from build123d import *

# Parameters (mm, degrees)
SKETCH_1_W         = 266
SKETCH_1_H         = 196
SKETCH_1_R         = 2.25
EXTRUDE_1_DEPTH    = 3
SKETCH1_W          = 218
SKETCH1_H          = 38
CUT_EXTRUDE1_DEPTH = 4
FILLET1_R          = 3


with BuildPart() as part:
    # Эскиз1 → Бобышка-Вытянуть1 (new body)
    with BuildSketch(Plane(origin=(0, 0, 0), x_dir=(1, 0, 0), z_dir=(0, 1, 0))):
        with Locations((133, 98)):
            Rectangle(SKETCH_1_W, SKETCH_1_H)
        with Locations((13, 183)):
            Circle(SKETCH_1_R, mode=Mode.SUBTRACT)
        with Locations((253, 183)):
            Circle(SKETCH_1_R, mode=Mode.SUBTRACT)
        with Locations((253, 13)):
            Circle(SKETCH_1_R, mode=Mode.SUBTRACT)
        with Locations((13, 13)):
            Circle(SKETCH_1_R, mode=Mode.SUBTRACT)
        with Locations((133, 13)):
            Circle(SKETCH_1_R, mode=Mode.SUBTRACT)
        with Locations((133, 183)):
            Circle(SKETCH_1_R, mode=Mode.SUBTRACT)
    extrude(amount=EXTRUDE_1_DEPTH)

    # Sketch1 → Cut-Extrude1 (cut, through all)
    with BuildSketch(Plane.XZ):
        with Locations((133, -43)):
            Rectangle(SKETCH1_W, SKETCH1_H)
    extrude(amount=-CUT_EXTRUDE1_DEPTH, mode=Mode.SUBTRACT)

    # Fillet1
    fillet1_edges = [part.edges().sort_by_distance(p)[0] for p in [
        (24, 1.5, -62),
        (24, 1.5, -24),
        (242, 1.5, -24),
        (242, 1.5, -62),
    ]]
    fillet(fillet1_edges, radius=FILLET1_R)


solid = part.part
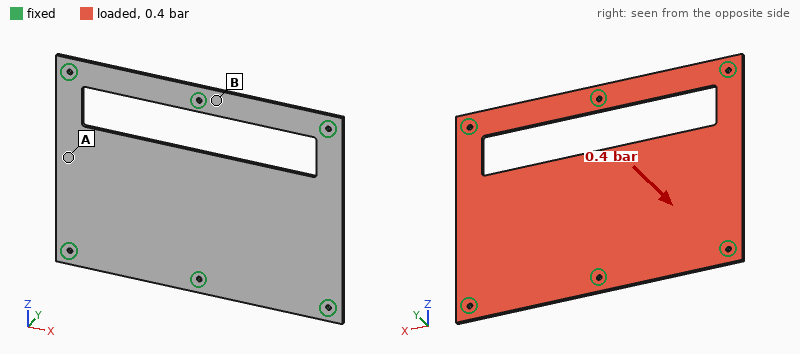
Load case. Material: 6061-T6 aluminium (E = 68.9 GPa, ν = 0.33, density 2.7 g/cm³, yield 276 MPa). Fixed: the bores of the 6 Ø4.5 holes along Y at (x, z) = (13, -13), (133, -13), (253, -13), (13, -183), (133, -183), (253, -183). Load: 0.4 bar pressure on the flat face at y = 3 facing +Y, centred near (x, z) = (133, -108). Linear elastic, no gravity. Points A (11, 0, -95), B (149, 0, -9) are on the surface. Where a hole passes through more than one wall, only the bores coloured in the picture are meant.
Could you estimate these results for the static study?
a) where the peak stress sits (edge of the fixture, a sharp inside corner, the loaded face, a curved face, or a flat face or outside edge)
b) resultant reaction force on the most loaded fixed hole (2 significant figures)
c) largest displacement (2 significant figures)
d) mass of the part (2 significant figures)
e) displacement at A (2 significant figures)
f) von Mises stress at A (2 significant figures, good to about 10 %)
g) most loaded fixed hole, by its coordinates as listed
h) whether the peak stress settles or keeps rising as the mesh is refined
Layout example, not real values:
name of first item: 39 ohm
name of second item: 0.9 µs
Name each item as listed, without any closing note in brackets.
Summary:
where the peak stress sits: edge of the fixture
resultant reaction force on the most loaded fixed hole: 590 N
largest displacement: 3.6 mm
mass of the part: 350 g
displacement at A: 1.1 mm
von Mises stress at A: 52 MPa
most loaded fixed hole, by its coordinates as listed: (133, -183)
whether the peak stress settles or keeps rising as the mesh is refined: keeps rising
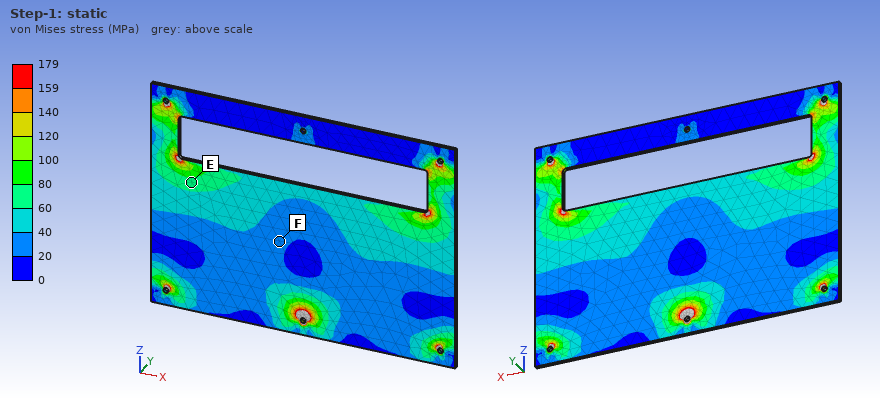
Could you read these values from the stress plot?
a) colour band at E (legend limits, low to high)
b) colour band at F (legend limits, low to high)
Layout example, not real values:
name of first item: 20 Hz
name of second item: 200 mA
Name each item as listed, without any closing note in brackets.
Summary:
colour band at E: 60 to 80 MPa
colour band at F: 20 to 40 MPa
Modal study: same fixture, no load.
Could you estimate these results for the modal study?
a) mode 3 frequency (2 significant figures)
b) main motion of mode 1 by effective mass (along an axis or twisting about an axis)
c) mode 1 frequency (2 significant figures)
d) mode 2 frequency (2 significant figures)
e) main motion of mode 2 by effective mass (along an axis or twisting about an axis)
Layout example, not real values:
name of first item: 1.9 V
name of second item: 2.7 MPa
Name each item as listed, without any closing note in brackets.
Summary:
mode 3 frequency: 610 Hz
main motion of mode 1 by effective mass: along Y
mode 1 frequency: 250 Hz
mode 2 frequency: 440 Hz
main motion of mode 2 by effective mass: twisting about Z
